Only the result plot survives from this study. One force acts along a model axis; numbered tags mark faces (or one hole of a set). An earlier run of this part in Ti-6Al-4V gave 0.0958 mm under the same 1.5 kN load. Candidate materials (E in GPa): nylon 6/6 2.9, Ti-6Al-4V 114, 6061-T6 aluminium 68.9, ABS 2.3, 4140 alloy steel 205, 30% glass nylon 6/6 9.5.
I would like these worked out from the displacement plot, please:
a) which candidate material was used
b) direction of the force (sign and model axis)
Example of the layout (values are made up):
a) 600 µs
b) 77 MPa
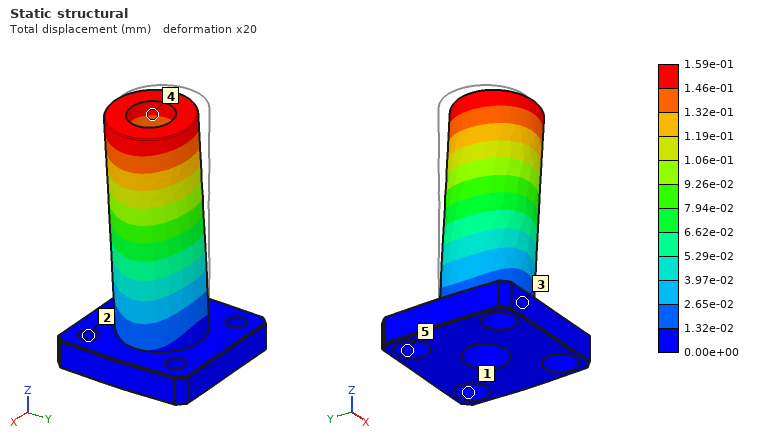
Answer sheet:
a) 6061-T6 aluminium
b) +X
